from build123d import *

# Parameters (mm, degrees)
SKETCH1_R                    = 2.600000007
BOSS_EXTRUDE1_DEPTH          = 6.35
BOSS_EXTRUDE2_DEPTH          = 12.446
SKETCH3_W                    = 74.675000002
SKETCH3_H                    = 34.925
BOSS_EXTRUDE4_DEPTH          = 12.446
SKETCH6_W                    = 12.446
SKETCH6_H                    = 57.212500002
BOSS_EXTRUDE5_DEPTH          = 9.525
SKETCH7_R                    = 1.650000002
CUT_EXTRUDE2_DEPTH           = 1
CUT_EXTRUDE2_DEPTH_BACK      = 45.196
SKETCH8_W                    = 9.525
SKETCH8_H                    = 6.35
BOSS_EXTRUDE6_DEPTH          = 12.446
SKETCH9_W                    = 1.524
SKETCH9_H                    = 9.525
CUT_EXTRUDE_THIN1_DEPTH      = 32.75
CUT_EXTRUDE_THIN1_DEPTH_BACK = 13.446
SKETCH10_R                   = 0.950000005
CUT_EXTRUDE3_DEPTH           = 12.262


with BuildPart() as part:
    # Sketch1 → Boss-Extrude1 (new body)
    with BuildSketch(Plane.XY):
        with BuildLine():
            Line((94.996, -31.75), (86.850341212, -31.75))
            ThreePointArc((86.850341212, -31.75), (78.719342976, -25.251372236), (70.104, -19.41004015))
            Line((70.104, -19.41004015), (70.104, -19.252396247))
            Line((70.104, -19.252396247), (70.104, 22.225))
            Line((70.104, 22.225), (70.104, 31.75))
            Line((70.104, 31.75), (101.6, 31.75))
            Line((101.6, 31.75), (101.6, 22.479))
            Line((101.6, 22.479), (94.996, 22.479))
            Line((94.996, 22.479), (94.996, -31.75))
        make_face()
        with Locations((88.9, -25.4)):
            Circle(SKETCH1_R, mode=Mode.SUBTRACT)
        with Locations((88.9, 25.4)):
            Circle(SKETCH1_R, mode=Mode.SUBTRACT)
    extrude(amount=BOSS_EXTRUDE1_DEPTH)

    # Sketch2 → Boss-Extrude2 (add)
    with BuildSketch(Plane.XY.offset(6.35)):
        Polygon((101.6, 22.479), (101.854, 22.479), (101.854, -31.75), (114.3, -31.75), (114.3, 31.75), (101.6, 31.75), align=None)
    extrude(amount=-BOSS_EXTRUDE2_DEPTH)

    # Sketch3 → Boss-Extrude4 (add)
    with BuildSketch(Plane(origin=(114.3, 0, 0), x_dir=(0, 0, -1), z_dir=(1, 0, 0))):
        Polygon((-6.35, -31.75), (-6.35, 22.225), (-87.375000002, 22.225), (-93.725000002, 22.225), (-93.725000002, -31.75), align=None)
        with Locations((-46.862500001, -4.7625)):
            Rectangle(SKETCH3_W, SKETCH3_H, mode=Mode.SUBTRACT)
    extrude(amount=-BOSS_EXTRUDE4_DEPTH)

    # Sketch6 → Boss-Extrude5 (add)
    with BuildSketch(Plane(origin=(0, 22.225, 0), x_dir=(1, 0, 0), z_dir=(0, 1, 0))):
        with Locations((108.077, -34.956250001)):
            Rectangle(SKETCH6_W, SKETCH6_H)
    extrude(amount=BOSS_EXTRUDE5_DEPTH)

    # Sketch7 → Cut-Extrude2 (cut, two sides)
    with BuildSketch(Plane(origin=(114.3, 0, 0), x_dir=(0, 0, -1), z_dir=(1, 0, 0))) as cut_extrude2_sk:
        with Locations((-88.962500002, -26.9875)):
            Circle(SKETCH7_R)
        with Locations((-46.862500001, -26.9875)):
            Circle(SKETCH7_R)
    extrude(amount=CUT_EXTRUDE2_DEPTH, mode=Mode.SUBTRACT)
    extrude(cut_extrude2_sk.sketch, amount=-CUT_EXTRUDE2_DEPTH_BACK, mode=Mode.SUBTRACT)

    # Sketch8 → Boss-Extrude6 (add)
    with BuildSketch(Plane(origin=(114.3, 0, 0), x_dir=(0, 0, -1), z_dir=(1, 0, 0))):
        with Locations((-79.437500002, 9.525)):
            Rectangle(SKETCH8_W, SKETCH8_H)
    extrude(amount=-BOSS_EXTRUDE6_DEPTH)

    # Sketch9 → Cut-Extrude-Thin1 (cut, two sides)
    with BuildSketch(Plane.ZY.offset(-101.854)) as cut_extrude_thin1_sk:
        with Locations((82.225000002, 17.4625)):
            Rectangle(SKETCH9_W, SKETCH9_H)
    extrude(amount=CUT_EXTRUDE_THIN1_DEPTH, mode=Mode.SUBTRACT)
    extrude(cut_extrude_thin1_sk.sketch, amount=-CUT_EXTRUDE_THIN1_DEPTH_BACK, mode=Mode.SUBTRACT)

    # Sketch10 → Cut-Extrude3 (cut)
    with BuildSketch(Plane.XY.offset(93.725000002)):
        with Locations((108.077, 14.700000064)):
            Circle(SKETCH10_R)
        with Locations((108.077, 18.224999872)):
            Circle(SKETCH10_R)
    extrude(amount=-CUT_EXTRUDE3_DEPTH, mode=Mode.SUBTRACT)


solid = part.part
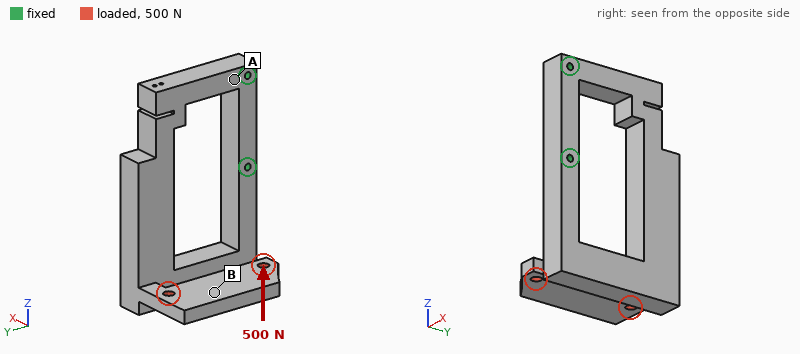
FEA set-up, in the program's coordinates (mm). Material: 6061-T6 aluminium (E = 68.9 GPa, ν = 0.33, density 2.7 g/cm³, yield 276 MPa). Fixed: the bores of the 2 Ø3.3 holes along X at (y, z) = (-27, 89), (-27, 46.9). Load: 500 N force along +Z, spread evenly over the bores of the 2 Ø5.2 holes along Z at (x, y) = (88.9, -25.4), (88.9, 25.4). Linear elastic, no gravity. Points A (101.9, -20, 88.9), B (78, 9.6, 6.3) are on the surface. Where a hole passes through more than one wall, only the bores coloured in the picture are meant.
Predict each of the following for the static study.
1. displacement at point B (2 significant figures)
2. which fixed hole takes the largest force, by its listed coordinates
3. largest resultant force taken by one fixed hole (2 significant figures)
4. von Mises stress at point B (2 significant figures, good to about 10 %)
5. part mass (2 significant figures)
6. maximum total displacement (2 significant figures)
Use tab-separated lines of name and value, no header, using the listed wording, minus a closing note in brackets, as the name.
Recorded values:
displacement at point B	0.51 mm
which fixed hole takes the largest force, by its listed coordinates	(-27, 46.9)
largest resultant force taken by one fixed hole	400 N
von Mises stress at point B	50 MPa
part mass	140 g
maximum total displacement	1.4 mm
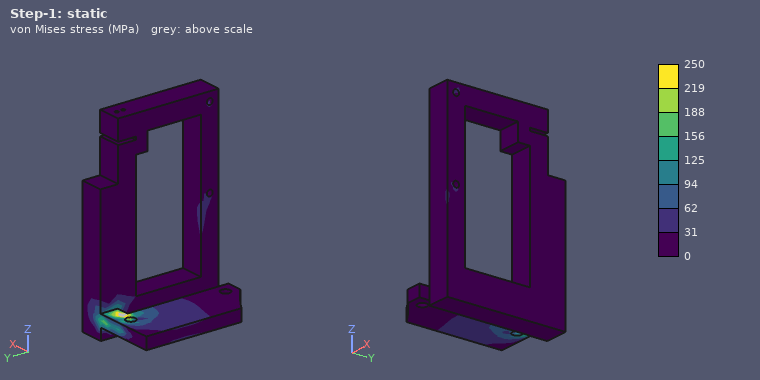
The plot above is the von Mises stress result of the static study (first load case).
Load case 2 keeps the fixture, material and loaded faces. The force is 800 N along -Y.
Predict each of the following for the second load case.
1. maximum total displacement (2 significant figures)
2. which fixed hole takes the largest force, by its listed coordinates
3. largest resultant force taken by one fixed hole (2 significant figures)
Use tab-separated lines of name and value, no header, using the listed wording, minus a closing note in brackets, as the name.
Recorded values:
maximum total displacement	0.71 mm
which fixed hole takes the largest force, by its listed coordinates	(-27, 46.9)
largest resultant force taken by one fixed hole	1.2 kN
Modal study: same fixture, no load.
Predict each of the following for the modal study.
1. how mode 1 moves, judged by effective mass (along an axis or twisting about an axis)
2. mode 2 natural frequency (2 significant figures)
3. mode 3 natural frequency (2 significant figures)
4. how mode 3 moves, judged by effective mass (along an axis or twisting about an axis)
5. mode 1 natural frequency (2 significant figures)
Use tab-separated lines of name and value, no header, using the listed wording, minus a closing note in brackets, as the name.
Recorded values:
how mode 1 moves, judged by effective mass	along X
mode 2 natural frequency	790 Hz
mode 3 natural frequency	950 Hz
how mode 3 moves, judged by effective mass	along Y
mode 1 natural frequency	600 Hz
